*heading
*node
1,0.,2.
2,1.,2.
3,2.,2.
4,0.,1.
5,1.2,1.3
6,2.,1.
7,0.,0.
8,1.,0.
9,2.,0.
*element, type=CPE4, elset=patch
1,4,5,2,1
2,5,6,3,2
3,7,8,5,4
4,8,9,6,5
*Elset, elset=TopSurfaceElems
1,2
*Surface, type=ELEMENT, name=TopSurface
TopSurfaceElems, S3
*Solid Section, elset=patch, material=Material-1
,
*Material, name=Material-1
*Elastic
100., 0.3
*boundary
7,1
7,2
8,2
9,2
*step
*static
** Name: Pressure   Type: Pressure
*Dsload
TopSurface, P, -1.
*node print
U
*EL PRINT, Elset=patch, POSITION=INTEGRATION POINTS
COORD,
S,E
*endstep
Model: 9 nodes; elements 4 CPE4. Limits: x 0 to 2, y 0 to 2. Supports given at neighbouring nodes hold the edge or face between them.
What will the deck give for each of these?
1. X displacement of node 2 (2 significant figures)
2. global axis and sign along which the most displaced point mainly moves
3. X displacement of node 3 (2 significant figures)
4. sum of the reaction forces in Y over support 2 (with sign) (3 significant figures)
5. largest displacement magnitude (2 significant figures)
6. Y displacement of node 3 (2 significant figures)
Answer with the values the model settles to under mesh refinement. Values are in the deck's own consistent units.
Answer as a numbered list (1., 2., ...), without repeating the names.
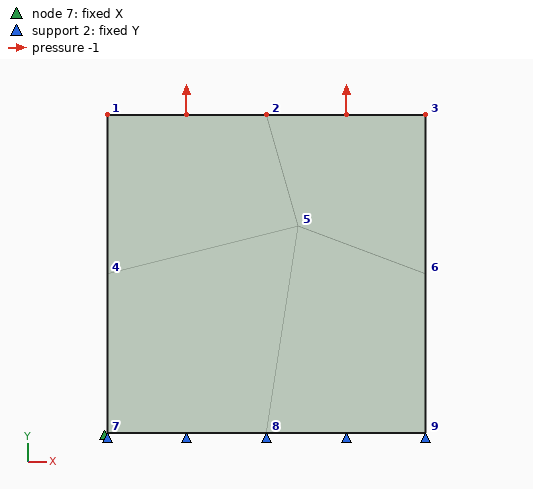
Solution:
1. -0.0039
2. +Y
3. -0.0078
4. -2.00
5. 0.020
6. 0.018
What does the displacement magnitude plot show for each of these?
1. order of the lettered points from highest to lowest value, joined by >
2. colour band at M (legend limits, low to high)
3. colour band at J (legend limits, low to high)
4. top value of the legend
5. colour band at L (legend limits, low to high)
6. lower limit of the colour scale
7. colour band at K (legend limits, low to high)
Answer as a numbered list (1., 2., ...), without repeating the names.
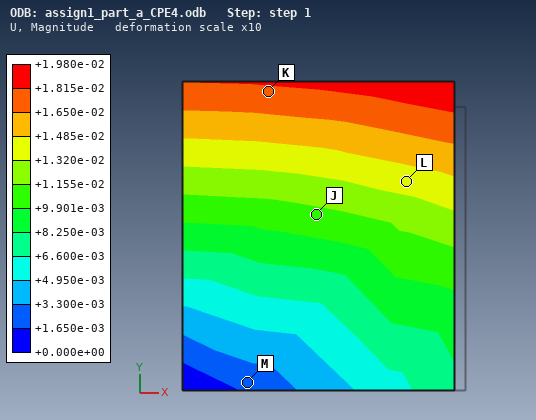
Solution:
1. K > L > J > M
2. +1.650e-03 to +3.300e-03
3. +9.901e-03 to +1.155e-02
4. +1.980e-02
5. +1.320e-02 to +1.485e-02
6. +0.000e+00
7. +1.650e-02 to +1.815e-02
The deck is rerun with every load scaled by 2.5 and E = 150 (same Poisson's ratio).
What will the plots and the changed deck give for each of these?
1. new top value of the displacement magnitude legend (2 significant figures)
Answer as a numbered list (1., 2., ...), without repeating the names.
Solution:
1. 0.033
